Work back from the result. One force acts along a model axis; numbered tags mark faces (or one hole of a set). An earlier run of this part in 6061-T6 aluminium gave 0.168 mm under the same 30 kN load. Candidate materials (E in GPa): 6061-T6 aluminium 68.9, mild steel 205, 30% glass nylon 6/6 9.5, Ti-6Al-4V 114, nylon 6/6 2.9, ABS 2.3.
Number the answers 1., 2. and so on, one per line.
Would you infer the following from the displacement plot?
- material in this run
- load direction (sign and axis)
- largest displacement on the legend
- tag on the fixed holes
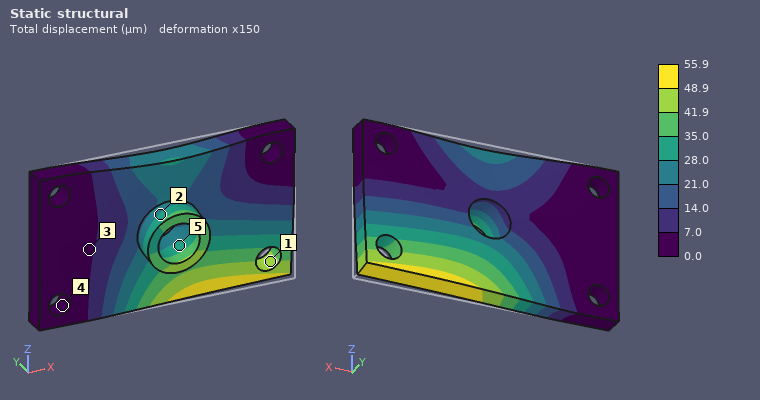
1. mild steel
2. -Z
3. 55.9 µm
4. 4
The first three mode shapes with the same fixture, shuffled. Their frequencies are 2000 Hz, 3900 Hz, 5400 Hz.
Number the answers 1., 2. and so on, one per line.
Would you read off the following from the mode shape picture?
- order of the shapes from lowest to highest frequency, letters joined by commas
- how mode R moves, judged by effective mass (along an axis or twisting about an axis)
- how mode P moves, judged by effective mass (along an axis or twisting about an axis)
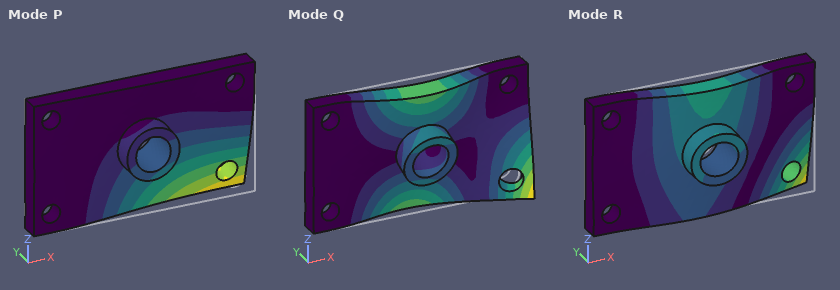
1. P, R, Q
2. along Y
3. along Y
